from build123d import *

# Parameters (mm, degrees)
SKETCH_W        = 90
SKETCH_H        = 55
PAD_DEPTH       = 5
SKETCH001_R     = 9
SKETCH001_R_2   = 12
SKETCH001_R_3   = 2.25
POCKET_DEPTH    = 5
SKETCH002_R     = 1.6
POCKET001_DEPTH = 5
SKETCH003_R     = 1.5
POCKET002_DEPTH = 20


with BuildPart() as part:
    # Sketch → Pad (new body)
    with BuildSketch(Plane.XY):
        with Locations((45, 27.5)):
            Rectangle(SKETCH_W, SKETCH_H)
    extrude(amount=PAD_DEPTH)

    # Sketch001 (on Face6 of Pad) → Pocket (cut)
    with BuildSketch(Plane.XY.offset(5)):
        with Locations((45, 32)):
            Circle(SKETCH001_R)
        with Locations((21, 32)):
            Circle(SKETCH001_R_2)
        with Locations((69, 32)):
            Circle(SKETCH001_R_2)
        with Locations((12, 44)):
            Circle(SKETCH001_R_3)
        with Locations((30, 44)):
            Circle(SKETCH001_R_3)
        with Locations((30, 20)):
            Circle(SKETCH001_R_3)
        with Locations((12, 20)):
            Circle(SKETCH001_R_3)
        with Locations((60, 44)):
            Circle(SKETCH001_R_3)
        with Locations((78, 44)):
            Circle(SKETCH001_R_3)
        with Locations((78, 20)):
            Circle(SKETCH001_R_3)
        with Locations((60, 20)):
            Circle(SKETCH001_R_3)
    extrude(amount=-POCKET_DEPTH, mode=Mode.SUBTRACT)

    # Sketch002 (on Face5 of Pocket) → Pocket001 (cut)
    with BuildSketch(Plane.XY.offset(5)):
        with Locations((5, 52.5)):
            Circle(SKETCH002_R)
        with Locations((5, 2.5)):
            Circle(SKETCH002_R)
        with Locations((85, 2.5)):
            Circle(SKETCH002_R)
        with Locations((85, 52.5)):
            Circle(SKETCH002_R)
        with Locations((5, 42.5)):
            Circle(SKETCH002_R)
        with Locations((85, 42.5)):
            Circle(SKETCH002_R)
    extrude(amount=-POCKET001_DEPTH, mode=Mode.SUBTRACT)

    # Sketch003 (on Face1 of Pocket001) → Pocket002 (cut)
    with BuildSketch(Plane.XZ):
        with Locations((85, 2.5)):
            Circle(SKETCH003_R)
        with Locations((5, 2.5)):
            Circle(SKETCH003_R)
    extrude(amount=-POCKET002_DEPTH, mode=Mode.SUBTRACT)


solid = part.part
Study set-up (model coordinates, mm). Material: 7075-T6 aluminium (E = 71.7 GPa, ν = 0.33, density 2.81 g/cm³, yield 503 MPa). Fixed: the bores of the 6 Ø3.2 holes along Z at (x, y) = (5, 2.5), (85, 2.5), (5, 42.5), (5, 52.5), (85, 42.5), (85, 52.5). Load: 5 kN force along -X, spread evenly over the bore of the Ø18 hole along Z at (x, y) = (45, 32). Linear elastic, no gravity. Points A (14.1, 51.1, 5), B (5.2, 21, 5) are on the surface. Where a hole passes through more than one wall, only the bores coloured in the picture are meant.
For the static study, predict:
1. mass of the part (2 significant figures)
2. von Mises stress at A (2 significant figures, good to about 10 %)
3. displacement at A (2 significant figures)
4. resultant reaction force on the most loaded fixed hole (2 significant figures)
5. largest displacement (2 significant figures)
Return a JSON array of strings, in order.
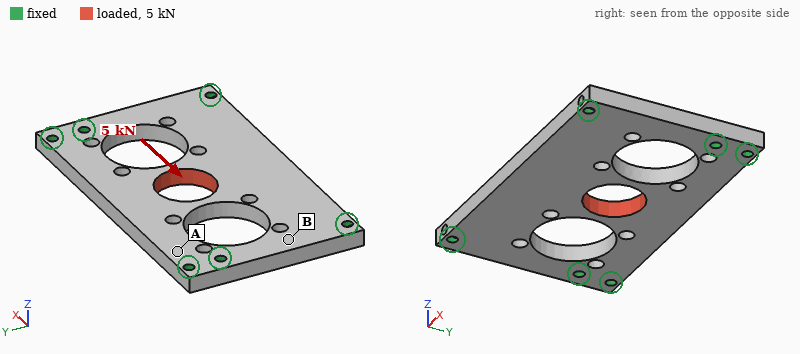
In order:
["50 g", "27 MPa", "4.6 µm", "1.3 kN", "28 µm"]
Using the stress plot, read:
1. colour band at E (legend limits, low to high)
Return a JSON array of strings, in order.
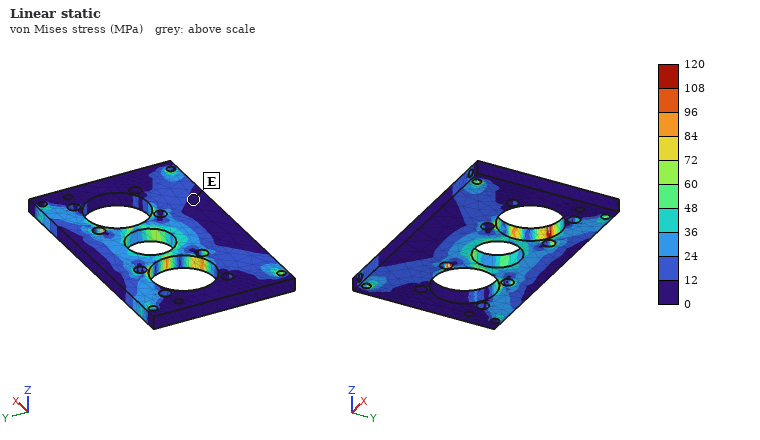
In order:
["0 to 12 MPa"]
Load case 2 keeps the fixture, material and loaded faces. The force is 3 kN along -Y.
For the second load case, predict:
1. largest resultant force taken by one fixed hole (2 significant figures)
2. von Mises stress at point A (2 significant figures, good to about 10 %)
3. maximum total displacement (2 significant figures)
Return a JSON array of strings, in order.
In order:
["1.2 kN", "19 MPa", "36 µm"]
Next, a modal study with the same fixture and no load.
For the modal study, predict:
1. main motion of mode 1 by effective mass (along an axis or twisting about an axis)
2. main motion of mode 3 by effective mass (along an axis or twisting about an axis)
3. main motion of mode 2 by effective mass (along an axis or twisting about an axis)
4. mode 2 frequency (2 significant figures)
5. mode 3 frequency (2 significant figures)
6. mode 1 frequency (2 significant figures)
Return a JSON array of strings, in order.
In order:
["along Z", "twisting about Y", "twisting about X", "4600 Hz", "8800 Hz", "3300 Hz"]
